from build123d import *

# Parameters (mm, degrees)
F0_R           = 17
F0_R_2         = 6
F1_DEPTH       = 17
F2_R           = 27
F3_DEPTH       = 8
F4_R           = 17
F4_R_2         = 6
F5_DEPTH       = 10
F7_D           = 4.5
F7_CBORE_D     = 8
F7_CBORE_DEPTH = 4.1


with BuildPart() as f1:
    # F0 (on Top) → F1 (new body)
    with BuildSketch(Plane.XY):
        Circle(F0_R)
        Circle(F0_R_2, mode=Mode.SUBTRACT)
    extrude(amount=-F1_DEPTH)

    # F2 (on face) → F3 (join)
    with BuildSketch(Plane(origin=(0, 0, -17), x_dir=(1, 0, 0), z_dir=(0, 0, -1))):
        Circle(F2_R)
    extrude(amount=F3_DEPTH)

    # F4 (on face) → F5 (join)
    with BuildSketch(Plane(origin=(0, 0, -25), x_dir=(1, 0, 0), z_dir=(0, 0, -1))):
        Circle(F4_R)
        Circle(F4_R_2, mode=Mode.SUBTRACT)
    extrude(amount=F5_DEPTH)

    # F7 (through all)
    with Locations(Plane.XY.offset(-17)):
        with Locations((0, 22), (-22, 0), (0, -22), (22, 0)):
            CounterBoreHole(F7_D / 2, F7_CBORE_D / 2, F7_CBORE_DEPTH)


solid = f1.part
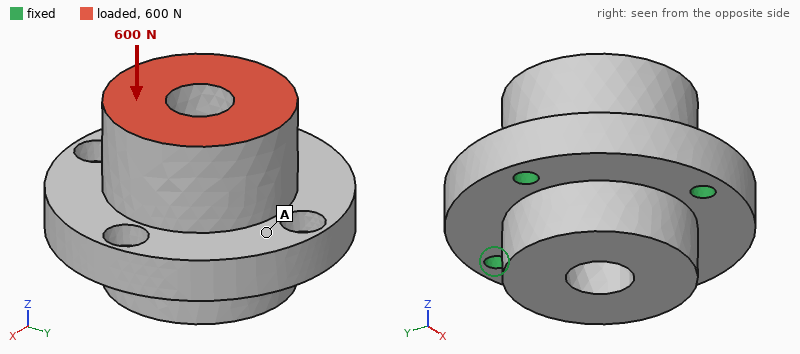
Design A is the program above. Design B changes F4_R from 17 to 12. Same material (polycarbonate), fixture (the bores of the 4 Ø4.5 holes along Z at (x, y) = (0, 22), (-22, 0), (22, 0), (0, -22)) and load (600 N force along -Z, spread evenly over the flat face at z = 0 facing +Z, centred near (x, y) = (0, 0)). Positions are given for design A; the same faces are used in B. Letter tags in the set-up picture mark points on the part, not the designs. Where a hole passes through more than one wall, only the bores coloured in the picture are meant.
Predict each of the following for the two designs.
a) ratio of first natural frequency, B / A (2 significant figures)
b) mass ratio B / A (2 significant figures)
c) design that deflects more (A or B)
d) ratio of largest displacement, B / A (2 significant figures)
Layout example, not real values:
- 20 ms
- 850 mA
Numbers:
- 1.00
- 0.88
- B
- 1.1
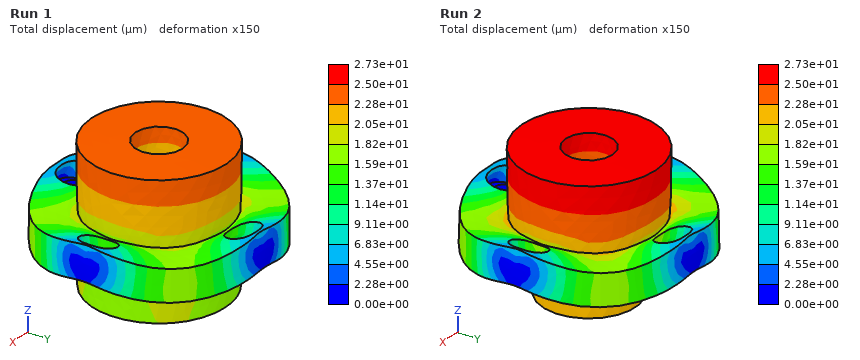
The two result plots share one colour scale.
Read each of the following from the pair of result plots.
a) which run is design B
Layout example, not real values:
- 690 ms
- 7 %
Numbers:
- Run 2
